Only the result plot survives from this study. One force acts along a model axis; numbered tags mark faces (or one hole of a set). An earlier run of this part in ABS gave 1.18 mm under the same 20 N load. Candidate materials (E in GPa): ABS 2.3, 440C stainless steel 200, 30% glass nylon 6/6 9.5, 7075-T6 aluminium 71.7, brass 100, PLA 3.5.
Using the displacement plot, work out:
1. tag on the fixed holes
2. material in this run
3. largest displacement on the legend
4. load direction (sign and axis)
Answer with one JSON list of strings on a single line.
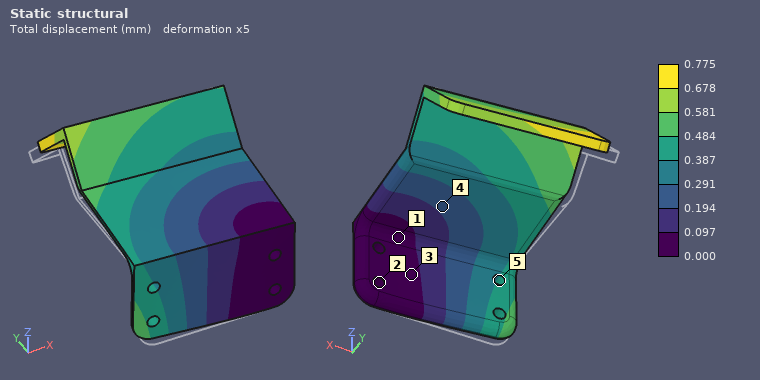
["2", "PLA", "0.775 mm", "+Y"]
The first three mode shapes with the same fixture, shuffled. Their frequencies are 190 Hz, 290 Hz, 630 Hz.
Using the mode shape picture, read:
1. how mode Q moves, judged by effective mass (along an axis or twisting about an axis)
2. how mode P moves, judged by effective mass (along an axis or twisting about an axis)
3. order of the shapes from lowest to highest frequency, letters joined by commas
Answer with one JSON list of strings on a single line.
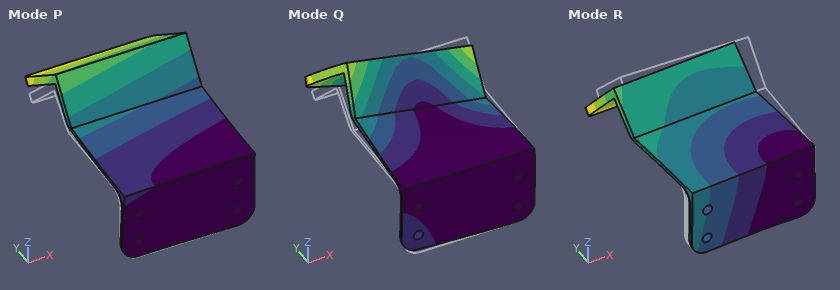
["twisting about Y", "along Z", "P, R, Q"]
